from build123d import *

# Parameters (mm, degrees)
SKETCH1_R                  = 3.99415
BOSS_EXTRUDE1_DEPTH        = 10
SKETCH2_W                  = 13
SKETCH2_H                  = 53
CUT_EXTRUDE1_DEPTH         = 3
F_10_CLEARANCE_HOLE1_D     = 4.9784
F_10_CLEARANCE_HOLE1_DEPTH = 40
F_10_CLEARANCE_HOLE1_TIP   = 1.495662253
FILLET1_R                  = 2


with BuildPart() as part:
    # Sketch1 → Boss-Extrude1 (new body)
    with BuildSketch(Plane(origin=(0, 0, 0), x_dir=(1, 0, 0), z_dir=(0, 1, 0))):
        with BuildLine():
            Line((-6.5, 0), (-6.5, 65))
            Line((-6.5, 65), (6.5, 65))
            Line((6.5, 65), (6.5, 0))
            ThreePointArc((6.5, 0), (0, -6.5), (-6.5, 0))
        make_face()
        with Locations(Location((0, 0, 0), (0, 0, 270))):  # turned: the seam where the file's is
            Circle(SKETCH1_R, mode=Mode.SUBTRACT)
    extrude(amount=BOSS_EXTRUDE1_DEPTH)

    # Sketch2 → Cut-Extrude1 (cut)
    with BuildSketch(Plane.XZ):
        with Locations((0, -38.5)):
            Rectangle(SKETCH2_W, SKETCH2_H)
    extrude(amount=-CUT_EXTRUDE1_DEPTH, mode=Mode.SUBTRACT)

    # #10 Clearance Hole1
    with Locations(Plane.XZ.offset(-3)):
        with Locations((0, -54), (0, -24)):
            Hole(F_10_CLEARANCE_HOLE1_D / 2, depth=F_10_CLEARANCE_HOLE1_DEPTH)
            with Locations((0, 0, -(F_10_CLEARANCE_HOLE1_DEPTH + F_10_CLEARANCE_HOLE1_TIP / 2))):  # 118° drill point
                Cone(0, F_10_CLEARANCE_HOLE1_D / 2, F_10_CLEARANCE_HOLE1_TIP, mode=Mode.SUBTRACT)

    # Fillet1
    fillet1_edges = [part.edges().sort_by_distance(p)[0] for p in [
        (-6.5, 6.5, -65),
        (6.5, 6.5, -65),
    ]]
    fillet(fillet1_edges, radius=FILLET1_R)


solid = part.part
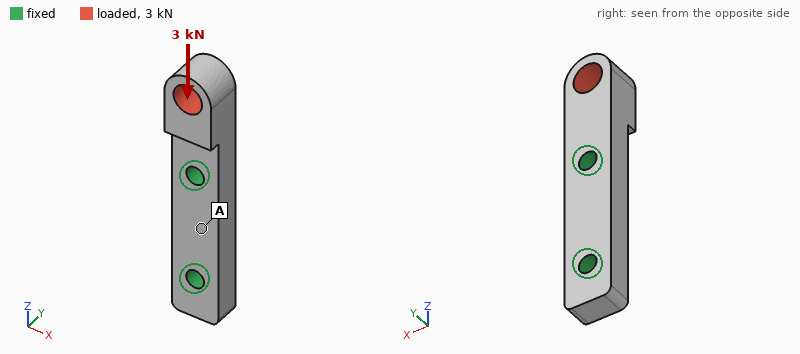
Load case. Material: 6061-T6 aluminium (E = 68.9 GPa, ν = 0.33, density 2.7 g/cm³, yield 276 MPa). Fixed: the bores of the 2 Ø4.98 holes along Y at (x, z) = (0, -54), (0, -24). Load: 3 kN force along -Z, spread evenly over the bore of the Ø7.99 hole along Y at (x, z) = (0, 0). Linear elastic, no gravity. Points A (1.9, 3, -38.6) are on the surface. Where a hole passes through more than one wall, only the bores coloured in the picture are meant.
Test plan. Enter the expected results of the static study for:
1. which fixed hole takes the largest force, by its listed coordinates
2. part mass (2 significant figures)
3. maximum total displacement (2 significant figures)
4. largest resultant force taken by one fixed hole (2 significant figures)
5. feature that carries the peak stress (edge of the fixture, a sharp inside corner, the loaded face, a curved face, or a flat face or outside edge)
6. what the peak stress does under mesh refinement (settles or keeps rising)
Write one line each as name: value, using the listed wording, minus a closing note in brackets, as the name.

which fixed hole takes the largest force, by its listed coordinates: (0, -24)
part mass: 17 g
maximum total displacement: 63 µm
largest resultant force taken by one fixed hole: 2.9 kN
feature that carries the peak stress: edge of the fixture
what the peak stress does under mesh refinement: keeps rising
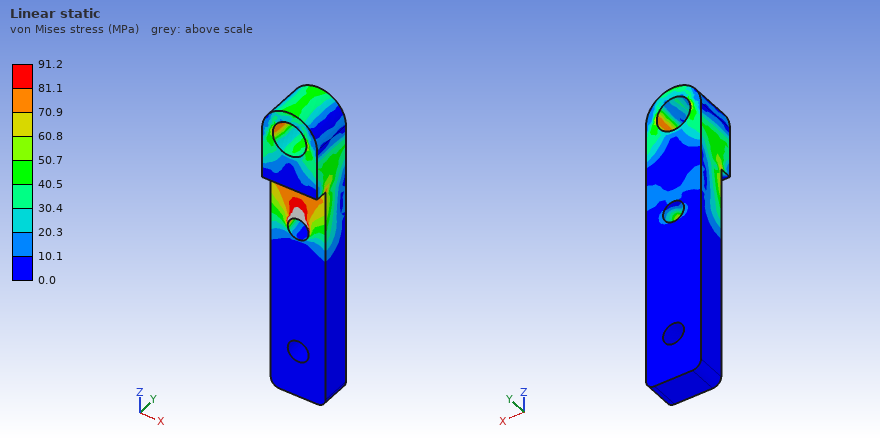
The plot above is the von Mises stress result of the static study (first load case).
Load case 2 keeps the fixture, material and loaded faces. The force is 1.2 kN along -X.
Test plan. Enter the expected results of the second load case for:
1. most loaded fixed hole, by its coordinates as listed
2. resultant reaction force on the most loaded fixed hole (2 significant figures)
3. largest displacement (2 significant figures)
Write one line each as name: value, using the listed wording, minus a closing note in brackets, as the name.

most loaded fixed hole, by its coordinates as listed: (0, -24)
resultant reaction force on the most loaded fixed hole: 1.5 kN
largest displacement: 0.14 mm
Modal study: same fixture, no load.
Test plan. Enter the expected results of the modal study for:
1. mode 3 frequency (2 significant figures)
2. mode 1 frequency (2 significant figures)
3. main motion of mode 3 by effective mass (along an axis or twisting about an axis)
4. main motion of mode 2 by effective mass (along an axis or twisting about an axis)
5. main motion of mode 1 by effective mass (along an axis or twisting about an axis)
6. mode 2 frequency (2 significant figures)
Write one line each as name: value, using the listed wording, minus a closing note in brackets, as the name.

mode 3 frequency: 20 kHz
mode 1 frequency: 7000 Hz
main motion of mode 3 by effective mass: twisting about Z
main motion of mode 2 by effective mass: along X
main motion of mode 1 by effective mass: along Y
mode 2 frequency: 9500 Hz
